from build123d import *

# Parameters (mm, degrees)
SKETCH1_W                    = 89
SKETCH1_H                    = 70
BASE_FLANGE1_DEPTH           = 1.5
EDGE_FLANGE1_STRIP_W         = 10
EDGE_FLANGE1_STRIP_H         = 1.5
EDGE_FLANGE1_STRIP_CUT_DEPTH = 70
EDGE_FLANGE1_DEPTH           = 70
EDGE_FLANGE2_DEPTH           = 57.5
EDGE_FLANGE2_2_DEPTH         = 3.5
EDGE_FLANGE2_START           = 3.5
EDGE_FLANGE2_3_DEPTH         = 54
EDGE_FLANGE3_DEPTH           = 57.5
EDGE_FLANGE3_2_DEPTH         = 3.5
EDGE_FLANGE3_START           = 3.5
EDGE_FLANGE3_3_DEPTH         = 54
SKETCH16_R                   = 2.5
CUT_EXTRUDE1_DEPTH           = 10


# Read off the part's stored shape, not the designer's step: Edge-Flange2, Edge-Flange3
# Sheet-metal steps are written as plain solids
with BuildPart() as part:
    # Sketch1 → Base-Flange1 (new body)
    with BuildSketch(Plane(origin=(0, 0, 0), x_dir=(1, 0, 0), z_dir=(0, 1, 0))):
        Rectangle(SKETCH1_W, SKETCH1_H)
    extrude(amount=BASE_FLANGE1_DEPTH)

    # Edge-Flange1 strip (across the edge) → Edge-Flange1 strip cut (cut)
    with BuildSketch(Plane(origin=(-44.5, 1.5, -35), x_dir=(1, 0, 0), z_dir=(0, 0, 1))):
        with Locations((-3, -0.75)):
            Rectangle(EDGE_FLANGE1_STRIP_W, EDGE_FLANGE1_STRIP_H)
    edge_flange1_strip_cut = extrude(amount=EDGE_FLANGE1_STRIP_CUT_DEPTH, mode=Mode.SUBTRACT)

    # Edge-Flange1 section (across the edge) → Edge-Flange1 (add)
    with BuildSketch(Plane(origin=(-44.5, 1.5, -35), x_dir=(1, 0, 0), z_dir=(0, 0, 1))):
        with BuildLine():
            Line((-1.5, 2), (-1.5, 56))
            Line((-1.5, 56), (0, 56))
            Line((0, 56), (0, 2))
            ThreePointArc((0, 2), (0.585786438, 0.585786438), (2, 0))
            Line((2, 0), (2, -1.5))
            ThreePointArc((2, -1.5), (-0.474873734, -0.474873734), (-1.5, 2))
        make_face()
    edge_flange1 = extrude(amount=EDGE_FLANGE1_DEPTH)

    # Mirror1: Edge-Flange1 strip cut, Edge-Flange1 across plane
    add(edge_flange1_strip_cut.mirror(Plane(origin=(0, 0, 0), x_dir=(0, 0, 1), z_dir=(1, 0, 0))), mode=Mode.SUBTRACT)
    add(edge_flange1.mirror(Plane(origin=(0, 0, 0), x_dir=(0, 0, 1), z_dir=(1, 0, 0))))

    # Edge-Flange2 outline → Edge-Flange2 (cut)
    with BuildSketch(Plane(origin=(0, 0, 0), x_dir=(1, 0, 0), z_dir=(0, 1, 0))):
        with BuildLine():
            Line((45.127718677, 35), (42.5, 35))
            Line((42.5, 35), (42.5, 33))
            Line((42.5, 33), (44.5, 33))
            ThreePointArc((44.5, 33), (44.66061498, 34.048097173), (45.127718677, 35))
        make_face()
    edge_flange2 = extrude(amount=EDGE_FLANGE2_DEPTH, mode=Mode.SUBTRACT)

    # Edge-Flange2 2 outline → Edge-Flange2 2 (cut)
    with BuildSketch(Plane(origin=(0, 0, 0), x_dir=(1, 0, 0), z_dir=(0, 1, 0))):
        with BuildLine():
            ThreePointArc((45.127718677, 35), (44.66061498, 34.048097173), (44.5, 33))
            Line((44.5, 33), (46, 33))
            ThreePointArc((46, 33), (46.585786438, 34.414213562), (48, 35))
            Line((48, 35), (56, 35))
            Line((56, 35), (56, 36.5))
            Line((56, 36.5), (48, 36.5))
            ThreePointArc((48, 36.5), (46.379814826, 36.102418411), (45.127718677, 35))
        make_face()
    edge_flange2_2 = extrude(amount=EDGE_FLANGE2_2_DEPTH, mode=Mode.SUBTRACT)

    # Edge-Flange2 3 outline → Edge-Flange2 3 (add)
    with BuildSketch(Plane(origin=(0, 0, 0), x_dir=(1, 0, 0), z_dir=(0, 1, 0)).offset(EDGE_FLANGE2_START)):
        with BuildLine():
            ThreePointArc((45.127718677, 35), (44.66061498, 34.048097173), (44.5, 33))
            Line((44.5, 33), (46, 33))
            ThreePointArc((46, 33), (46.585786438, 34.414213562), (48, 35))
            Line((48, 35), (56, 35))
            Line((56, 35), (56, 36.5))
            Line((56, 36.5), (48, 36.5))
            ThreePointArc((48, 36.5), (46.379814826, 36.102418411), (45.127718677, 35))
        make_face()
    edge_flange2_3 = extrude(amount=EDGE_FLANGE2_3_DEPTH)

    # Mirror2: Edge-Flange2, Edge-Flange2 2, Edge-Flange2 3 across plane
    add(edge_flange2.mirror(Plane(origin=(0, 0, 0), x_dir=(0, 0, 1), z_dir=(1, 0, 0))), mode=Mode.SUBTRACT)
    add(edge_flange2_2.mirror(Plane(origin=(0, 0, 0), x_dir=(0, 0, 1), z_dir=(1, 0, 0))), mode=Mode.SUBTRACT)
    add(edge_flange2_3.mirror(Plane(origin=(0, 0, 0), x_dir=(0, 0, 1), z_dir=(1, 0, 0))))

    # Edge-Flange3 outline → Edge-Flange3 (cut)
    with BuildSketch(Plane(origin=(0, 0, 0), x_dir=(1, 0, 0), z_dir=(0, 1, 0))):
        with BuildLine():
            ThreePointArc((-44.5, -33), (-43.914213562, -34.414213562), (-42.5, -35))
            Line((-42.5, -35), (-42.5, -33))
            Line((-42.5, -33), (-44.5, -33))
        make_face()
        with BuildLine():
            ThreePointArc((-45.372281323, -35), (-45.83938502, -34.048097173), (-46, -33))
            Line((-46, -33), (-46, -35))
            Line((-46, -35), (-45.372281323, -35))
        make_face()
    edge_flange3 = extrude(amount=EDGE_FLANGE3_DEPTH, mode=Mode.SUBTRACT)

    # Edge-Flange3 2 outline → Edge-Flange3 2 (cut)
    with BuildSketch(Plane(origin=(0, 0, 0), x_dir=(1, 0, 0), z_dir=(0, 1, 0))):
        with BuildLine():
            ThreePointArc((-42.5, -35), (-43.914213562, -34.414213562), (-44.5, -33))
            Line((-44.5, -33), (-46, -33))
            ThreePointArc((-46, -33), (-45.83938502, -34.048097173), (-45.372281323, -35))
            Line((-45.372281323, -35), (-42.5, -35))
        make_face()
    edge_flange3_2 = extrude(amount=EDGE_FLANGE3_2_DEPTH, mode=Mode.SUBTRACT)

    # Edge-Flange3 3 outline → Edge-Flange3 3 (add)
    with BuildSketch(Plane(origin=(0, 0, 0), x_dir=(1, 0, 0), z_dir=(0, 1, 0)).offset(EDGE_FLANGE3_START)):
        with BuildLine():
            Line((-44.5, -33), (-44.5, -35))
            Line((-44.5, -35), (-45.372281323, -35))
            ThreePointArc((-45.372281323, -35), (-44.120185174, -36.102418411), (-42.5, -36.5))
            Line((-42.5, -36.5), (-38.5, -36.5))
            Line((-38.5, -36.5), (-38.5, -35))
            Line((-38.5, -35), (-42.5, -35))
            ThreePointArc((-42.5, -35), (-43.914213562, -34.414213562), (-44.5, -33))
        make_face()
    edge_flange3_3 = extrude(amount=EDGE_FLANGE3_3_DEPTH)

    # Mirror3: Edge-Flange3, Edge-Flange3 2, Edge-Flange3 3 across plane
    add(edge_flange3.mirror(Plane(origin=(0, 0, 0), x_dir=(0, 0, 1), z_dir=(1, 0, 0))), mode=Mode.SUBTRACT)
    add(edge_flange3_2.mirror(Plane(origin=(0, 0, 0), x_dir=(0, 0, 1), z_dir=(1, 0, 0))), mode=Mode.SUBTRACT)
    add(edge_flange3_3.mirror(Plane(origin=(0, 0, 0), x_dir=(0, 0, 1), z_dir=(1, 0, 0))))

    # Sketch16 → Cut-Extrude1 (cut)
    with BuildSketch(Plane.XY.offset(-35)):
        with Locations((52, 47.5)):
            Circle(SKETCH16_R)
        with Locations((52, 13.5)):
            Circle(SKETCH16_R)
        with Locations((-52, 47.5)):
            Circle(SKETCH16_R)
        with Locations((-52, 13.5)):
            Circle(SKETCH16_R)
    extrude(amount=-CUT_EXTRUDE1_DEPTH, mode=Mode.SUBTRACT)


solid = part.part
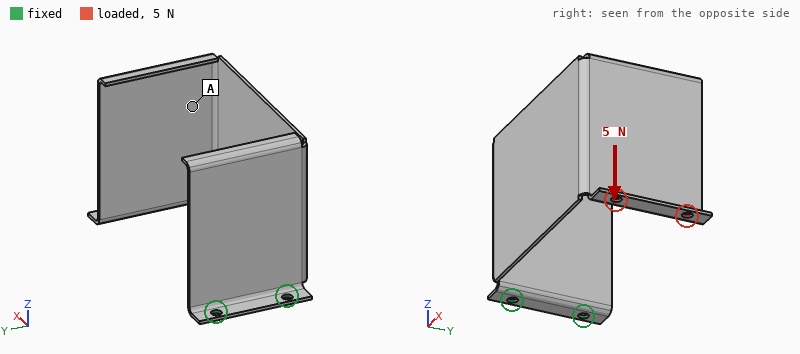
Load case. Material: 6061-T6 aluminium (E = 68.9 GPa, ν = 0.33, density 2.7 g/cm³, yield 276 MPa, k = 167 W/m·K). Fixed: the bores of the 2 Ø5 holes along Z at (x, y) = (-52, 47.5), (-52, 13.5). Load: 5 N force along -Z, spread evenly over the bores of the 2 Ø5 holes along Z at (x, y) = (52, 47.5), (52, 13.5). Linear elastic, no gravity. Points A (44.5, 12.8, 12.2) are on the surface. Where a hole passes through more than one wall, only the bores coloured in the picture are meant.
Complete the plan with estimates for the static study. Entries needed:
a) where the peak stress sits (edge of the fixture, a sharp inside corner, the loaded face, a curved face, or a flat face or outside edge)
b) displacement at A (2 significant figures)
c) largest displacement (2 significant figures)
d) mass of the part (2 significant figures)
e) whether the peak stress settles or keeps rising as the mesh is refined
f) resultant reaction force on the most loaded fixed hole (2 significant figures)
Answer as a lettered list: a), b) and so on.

a) a sharp inside corner
b) 1.3 mm
c) 1.6 mm
d) 64 g
e) keeps rising
f) 9.2 N
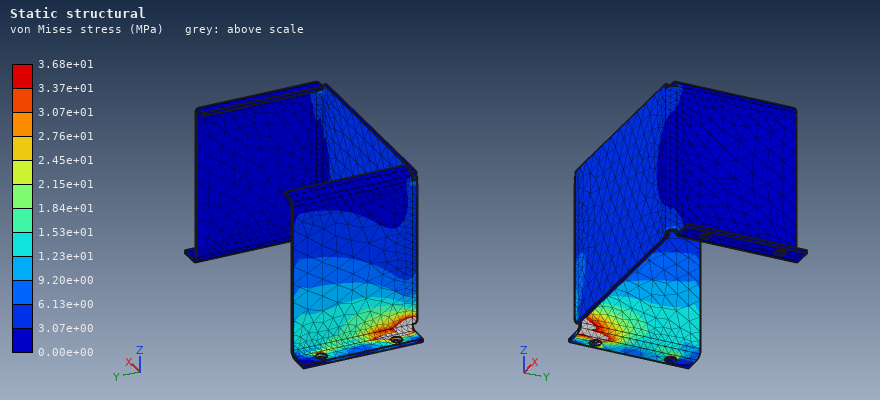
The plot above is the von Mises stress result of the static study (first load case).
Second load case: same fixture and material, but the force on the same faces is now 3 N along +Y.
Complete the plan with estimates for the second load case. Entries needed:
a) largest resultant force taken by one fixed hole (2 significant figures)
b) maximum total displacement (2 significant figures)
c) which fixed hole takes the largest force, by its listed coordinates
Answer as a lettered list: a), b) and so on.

a) 10 N
b) 1.5 mm
c) (-52, 47.5)
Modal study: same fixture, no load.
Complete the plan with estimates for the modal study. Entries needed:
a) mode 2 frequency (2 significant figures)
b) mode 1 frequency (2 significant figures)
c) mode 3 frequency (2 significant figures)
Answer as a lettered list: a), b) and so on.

a) 62 Hz
b) 50 Hz
c) 160 Hz
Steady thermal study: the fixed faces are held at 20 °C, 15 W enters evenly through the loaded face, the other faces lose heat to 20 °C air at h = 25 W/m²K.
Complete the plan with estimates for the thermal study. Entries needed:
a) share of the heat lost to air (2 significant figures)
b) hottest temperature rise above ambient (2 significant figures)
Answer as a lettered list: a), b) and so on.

a) 89 %
b) 70 K
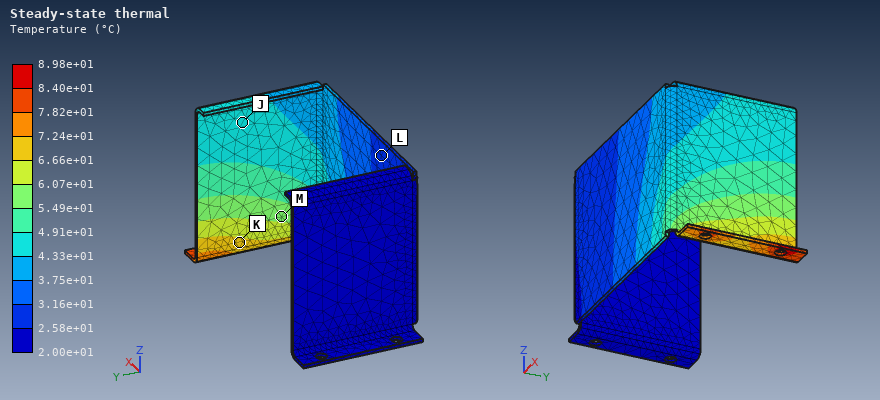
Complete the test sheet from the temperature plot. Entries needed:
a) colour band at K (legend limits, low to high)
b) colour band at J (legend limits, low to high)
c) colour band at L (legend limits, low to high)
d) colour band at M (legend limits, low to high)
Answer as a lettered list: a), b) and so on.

a) 6.66e+01 to 7.24e+01 °C
b) 4.33e+01 to 4.91e+01 °C
c) 2.58e+01 to 3.16e+01 °C
d) 5.49e+01 to 6.07e+01 °C
